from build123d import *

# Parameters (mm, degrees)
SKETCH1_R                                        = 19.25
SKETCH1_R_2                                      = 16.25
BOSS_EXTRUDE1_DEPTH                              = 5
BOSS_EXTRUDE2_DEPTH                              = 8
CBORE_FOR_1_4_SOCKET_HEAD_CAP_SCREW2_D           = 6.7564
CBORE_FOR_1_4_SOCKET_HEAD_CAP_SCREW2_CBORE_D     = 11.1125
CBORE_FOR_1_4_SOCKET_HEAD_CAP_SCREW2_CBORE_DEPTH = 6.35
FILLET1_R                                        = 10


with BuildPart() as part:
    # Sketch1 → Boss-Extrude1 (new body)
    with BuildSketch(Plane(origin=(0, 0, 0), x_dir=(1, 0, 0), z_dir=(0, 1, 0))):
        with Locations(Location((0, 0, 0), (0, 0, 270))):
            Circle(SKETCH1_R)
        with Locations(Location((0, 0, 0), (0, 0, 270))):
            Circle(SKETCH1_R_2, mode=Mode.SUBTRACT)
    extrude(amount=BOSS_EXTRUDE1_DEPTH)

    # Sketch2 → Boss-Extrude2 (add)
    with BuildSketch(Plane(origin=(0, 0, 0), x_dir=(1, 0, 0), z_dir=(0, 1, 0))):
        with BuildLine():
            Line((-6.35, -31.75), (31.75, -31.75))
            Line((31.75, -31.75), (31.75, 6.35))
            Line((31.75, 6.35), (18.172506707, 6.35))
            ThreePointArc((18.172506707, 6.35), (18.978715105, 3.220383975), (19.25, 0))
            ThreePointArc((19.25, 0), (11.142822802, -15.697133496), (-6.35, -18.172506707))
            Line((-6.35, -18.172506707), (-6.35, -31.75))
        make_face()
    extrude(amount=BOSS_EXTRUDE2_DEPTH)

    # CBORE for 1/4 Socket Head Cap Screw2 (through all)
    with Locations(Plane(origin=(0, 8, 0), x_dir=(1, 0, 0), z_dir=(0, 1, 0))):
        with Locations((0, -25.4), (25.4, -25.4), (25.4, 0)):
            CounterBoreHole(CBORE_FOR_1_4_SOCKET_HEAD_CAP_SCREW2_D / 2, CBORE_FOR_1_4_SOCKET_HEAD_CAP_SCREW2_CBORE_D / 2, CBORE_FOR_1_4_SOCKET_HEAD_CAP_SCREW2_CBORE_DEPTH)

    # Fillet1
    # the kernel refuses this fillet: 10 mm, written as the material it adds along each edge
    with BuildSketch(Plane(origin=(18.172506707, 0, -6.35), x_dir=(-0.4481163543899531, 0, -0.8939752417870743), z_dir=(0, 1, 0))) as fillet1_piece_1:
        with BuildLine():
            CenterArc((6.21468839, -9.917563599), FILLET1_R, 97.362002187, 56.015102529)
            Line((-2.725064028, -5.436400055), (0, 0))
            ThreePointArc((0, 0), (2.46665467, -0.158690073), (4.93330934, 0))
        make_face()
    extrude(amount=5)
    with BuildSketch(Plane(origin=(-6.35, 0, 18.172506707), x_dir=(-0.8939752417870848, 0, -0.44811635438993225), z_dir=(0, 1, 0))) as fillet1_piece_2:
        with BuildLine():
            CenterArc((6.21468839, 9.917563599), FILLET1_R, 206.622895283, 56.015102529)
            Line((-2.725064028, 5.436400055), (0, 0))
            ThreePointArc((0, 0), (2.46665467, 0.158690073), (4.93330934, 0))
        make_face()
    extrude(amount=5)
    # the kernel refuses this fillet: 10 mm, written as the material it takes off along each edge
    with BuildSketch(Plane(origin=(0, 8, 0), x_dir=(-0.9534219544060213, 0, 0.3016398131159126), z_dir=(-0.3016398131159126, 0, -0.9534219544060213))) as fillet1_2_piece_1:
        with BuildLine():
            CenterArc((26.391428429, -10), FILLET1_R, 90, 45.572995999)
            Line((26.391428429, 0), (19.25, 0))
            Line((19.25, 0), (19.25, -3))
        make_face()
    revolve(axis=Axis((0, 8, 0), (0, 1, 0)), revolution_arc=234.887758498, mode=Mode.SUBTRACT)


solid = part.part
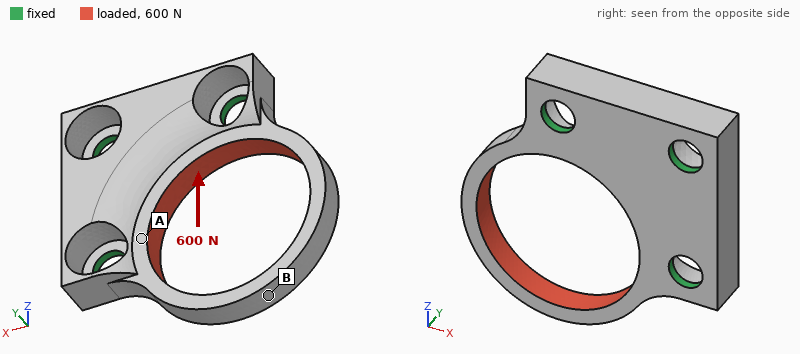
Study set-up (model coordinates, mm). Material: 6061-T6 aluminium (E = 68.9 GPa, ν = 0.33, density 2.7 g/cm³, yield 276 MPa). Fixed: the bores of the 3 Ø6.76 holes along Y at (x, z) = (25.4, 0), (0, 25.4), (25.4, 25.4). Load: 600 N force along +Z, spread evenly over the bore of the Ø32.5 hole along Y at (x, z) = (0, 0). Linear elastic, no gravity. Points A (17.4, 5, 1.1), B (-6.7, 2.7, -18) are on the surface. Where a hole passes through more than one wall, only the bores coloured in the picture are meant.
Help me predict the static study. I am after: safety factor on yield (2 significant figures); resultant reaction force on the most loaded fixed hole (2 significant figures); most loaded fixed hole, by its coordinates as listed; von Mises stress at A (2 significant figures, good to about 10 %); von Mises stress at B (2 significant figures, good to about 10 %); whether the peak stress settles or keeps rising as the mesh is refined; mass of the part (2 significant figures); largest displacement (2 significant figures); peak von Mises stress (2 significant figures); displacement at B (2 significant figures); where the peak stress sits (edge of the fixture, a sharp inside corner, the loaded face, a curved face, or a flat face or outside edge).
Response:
2.2
410 N
(0, 25.4)
17 MPa
54 MPa
settles
18 g
0.13 mm
130 MPa
0.12 mm
a curved face
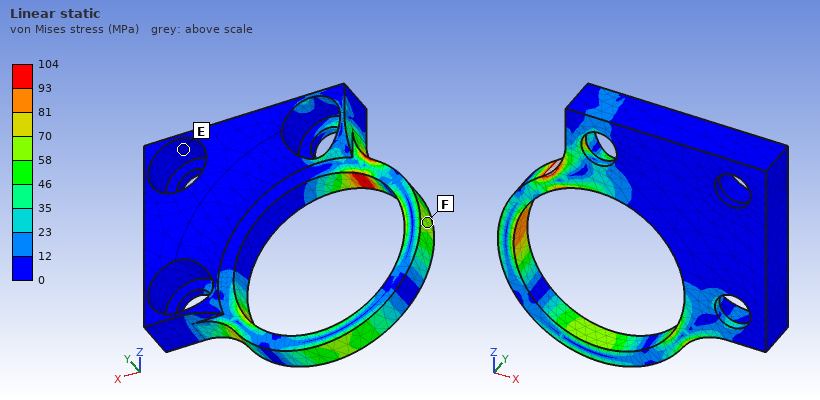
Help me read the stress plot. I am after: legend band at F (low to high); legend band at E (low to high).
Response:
58 to 70 MPa
0 to 12 MPa
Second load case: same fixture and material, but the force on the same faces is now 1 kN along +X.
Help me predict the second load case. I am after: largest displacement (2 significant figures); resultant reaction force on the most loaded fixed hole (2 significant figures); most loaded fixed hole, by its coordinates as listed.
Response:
0.22 mm
680 N
(25.4, 0)
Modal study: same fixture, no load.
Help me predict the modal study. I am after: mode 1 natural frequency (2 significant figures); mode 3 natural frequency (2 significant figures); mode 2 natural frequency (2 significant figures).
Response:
2600 Hz
6500 Hz
4700 Hz
